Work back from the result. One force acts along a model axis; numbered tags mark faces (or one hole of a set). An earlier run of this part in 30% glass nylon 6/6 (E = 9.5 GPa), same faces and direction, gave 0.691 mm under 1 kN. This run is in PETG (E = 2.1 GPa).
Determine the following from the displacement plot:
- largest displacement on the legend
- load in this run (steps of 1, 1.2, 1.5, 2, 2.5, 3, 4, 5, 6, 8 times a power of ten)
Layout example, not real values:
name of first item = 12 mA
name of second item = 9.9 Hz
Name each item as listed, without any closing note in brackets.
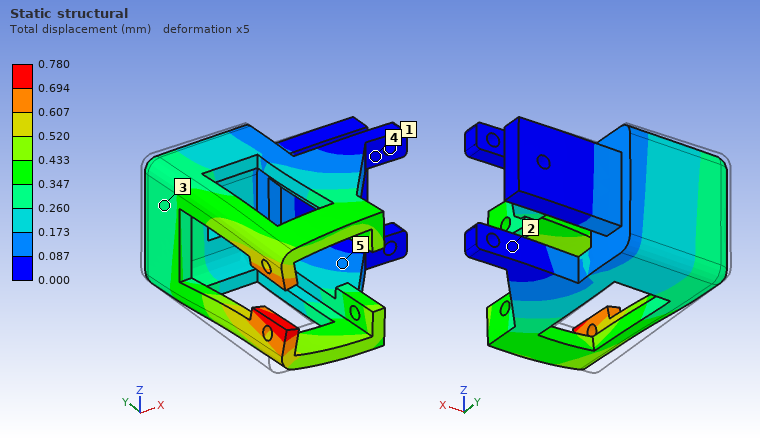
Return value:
largest displacement on the legend = 0.780 mm
load in this run = 250 N
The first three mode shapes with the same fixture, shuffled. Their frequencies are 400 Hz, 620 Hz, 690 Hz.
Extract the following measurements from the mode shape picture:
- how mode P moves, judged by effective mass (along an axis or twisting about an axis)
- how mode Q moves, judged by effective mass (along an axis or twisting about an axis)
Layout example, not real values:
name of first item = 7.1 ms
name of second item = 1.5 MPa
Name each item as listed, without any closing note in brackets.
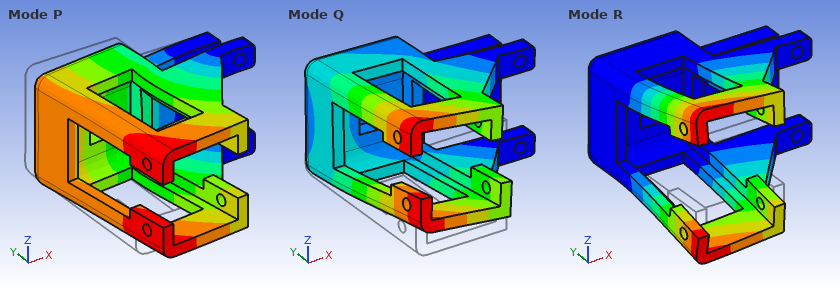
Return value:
how mode P moves, judged by effective mass = along Y
how mode Q moves, judged by effective mass = along Z
